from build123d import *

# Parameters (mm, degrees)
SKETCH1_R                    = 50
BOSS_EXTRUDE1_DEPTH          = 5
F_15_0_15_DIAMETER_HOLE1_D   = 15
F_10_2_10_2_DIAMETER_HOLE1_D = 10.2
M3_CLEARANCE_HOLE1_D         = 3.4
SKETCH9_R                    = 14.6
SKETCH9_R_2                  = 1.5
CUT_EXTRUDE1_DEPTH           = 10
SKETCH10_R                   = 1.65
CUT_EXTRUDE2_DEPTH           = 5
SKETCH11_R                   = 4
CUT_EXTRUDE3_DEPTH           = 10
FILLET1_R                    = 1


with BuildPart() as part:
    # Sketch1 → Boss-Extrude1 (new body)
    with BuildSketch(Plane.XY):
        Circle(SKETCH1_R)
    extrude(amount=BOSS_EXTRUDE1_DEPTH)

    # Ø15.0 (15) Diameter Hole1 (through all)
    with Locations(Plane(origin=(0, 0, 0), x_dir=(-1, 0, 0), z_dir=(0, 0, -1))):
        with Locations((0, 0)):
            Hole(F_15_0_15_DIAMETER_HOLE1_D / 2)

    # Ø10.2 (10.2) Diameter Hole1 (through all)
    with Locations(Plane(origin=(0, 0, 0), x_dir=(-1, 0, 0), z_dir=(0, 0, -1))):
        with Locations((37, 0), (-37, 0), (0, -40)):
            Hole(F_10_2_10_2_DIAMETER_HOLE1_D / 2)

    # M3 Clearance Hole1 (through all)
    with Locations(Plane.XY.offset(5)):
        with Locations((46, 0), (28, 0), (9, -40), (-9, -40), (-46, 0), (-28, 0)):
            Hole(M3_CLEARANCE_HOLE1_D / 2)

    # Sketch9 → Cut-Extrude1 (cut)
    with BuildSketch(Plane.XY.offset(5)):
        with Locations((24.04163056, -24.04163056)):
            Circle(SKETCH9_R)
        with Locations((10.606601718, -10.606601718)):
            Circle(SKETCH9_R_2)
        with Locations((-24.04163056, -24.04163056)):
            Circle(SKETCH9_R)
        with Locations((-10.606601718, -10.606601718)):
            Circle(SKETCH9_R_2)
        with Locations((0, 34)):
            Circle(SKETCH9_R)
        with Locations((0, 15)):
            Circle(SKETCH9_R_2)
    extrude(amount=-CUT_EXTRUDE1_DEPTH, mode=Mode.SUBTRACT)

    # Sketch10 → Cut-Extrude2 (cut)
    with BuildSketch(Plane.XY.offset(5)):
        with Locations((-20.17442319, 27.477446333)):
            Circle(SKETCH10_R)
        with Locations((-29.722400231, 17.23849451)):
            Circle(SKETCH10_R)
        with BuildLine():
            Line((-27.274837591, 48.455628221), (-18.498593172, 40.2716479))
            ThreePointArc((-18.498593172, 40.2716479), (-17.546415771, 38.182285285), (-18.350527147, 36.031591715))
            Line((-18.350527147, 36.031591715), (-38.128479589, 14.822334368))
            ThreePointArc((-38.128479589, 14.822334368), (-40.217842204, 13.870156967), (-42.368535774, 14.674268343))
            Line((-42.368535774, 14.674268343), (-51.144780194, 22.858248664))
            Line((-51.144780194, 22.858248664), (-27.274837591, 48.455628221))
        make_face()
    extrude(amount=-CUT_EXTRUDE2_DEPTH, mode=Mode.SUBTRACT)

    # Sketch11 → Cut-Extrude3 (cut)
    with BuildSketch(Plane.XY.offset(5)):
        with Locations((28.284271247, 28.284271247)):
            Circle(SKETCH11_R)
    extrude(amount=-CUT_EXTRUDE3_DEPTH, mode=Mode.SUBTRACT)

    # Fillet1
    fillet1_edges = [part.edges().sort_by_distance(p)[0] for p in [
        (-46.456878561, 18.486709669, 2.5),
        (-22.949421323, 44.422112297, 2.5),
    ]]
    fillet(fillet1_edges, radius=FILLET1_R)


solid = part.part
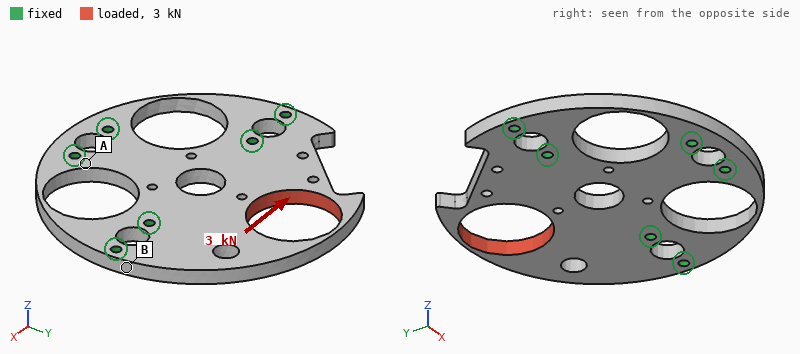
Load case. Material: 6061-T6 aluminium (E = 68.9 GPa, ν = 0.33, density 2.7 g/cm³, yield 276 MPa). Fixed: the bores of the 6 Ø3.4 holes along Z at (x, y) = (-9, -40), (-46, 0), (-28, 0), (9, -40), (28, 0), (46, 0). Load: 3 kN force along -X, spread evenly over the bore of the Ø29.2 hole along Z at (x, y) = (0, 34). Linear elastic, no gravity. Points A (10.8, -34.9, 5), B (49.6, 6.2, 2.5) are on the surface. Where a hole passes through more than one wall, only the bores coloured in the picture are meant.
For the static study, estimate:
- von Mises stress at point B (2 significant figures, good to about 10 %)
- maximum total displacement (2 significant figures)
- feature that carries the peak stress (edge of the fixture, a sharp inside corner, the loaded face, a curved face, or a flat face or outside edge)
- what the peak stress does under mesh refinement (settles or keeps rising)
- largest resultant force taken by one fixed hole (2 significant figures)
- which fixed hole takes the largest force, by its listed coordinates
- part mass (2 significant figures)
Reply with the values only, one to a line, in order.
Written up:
24 MPa
80 µm
a sharp inside corner
keeps rising
1.5 kN
(46, 0)
66 g
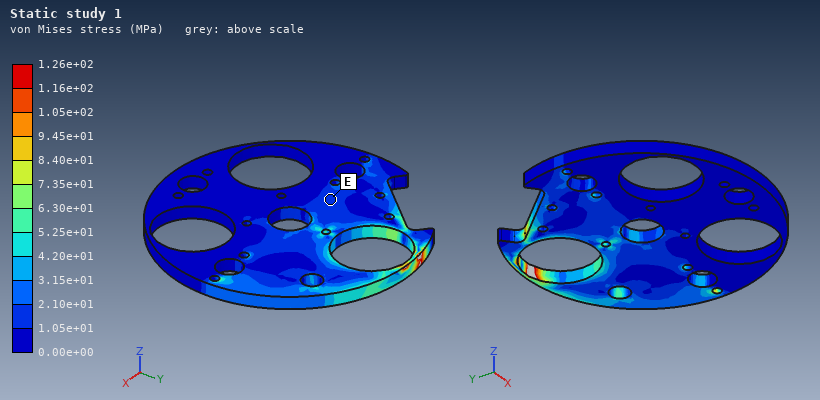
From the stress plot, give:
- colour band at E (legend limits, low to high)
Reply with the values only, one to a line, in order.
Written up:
1.05e+01 to 2.10e+01 MPa
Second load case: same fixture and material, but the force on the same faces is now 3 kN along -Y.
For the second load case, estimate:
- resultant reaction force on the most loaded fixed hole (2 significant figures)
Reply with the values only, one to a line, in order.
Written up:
1.2 kN
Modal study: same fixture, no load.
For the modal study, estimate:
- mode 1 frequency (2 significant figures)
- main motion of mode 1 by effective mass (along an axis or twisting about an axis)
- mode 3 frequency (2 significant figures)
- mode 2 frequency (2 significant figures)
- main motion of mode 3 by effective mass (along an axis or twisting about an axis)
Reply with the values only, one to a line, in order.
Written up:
2200 Hz
along Z
6900 Hz
4100 Hz
along Z
